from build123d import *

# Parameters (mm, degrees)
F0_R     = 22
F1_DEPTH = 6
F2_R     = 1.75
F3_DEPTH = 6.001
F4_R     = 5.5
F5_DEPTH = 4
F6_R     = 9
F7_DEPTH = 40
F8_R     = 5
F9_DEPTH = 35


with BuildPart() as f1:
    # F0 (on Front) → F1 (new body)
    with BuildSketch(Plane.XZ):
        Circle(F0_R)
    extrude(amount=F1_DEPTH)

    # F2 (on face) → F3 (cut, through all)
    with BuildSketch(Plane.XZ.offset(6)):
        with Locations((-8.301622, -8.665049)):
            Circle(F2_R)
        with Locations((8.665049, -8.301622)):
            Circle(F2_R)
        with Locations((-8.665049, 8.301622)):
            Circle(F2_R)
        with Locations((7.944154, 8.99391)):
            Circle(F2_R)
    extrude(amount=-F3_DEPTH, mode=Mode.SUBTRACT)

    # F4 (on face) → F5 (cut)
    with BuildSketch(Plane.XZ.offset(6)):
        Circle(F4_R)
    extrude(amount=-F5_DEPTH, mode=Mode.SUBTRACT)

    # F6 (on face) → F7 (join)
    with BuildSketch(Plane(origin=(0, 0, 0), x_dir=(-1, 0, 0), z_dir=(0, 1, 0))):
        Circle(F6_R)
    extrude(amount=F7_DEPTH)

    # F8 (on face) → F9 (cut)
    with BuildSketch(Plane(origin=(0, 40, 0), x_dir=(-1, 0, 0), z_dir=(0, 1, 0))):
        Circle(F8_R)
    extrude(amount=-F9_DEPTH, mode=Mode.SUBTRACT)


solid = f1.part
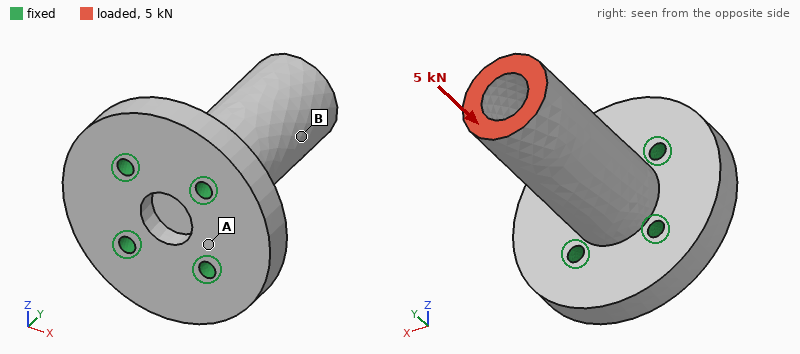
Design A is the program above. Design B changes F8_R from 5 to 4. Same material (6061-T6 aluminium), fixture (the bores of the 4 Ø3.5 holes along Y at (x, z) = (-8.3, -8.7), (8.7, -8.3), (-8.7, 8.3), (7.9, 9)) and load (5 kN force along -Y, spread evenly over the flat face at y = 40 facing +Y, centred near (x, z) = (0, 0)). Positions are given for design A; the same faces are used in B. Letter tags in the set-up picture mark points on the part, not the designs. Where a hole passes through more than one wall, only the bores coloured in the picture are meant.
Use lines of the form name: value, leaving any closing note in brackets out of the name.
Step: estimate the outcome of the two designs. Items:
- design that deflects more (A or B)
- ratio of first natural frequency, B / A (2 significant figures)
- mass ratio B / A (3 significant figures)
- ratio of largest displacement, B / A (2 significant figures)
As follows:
design that deflects more: A
ratio of first natural frequency, B / A: 0.96
mass ratio B / A: 1.06
ratio of largest displacement, B / A: 0.90
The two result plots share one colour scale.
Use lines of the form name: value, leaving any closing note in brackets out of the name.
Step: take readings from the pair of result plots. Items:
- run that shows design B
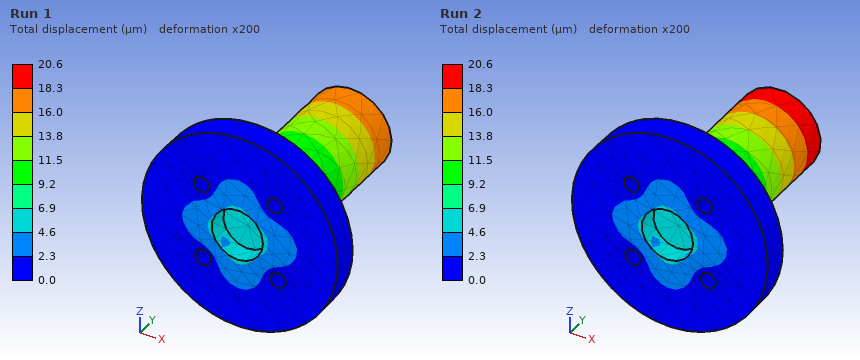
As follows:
run that shows design B: Run 1
